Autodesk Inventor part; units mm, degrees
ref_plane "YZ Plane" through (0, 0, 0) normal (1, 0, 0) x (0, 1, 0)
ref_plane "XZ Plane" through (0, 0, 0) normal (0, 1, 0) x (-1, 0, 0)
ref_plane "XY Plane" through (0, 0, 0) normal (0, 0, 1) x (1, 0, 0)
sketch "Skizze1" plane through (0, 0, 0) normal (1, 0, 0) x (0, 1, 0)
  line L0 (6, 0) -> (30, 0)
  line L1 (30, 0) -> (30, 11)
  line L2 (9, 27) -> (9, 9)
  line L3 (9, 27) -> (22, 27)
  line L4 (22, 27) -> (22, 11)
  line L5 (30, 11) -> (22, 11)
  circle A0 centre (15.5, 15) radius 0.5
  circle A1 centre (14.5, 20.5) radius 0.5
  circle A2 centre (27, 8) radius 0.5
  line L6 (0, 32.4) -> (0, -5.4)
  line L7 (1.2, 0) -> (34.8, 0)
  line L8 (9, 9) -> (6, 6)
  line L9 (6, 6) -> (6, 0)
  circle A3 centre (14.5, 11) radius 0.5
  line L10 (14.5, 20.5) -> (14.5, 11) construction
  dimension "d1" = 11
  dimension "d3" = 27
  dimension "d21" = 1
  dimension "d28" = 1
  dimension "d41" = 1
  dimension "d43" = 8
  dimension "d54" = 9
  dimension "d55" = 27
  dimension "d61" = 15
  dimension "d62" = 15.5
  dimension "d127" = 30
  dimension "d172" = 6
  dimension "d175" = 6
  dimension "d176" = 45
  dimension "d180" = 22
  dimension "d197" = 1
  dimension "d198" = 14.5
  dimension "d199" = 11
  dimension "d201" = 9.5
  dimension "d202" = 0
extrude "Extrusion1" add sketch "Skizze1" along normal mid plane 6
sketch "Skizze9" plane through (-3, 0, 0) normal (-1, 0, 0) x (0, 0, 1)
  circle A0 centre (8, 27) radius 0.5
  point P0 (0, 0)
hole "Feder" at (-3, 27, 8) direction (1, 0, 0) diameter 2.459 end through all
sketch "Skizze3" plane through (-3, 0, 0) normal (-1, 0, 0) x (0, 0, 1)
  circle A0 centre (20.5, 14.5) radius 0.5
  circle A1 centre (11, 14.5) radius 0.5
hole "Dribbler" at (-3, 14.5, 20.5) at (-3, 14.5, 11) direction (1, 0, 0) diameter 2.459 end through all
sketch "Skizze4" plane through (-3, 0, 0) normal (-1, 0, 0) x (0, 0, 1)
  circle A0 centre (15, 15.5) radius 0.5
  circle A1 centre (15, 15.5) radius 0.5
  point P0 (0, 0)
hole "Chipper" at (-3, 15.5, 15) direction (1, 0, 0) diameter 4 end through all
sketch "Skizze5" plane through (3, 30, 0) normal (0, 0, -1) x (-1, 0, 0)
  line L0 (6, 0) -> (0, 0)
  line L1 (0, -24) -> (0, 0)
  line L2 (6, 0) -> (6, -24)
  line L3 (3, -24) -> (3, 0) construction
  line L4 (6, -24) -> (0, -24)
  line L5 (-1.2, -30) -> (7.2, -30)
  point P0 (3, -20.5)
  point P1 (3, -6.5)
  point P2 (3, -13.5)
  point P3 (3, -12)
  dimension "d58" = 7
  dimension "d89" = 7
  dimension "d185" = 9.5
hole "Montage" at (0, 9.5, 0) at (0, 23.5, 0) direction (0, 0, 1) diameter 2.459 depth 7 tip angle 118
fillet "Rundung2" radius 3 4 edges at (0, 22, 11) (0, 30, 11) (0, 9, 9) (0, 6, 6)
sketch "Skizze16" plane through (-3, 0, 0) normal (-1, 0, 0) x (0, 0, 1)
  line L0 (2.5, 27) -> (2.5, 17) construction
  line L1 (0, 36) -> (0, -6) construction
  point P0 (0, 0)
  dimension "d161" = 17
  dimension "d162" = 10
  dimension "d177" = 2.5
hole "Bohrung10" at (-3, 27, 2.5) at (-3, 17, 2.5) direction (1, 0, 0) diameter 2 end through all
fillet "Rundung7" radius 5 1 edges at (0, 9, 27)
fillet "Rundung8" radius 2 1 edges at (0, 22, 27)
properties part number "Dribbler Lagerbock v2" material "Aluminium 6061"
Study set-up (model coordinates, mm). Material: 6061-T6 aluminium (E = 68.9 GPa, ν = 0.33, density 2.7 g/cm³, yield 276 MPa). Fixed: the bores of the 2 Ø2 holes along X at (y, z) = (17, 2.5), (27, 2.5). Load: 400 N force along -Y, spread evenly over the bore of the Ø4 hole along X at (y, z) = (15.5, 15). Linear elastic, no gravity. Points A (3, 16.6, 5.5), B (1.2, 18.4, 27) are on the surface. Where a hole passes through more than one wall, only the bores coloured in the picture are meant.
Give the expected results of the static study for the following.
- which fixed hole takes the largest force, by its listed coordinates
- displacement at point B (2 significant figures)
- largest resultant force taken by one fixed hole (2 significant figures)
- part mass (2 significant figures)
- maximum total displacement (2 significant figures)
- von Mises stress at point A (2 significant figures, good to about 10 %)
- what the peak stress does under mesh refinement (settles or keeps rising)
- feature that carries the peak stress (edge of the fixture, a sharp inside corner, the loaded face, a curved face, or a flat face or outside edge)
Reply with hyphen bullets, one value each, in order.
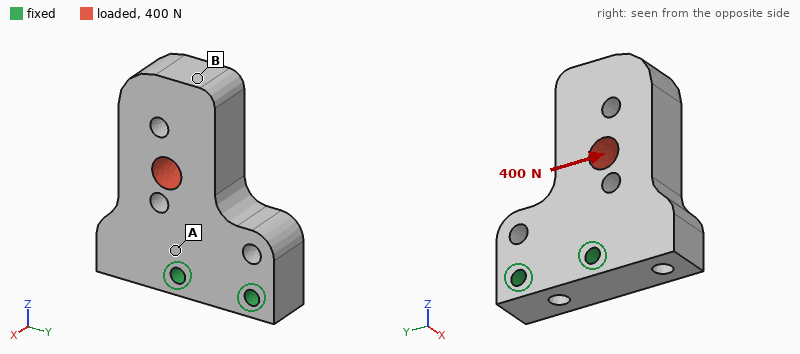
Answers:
- (27, 2.5)
- 13 µm
- 490 N
- 6.7 g
- 13 µm
- 13 MPa
- keeps rising
- edge of the fixture
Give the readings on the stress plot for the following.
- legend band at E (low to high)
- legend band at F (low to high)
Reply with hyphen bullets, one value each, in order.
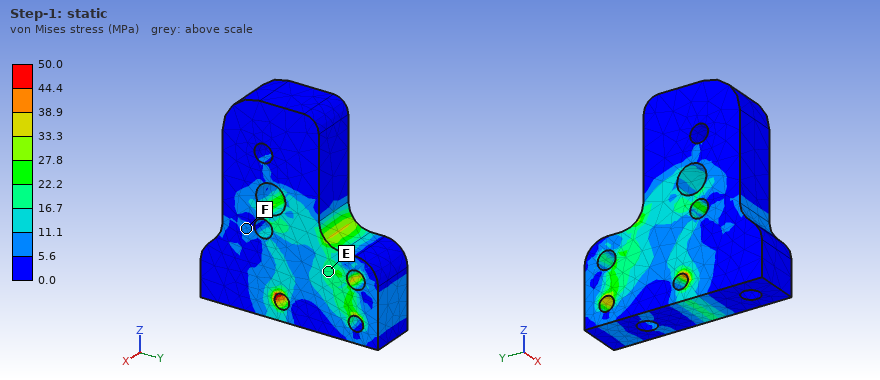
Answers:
- 16.7 to 22.2 MPa
- 5.6 to 11.1 MPa
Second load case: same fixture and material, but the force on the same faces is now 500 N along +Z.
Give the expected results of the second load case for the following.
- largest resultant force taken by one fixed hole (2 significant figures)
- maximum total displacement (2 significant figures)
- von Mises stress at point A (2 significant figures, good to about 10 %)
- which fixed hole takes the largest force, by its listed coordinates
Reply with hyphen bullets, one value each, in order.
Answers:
- 530 N
- 5.6 µm
- 14 MPa
- (17, 2.5)
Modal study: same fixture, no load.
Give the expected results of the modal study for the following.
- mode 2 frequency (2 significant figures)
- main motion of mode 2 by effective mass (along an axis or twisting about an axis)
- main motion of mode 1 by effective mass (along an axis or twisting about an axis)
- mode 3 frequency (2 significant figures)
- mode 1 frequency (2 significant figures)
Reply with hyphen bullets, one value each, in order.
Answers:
- 14 kHz
- along Y
- along X
- 22 kHz
- 7800 Hz
